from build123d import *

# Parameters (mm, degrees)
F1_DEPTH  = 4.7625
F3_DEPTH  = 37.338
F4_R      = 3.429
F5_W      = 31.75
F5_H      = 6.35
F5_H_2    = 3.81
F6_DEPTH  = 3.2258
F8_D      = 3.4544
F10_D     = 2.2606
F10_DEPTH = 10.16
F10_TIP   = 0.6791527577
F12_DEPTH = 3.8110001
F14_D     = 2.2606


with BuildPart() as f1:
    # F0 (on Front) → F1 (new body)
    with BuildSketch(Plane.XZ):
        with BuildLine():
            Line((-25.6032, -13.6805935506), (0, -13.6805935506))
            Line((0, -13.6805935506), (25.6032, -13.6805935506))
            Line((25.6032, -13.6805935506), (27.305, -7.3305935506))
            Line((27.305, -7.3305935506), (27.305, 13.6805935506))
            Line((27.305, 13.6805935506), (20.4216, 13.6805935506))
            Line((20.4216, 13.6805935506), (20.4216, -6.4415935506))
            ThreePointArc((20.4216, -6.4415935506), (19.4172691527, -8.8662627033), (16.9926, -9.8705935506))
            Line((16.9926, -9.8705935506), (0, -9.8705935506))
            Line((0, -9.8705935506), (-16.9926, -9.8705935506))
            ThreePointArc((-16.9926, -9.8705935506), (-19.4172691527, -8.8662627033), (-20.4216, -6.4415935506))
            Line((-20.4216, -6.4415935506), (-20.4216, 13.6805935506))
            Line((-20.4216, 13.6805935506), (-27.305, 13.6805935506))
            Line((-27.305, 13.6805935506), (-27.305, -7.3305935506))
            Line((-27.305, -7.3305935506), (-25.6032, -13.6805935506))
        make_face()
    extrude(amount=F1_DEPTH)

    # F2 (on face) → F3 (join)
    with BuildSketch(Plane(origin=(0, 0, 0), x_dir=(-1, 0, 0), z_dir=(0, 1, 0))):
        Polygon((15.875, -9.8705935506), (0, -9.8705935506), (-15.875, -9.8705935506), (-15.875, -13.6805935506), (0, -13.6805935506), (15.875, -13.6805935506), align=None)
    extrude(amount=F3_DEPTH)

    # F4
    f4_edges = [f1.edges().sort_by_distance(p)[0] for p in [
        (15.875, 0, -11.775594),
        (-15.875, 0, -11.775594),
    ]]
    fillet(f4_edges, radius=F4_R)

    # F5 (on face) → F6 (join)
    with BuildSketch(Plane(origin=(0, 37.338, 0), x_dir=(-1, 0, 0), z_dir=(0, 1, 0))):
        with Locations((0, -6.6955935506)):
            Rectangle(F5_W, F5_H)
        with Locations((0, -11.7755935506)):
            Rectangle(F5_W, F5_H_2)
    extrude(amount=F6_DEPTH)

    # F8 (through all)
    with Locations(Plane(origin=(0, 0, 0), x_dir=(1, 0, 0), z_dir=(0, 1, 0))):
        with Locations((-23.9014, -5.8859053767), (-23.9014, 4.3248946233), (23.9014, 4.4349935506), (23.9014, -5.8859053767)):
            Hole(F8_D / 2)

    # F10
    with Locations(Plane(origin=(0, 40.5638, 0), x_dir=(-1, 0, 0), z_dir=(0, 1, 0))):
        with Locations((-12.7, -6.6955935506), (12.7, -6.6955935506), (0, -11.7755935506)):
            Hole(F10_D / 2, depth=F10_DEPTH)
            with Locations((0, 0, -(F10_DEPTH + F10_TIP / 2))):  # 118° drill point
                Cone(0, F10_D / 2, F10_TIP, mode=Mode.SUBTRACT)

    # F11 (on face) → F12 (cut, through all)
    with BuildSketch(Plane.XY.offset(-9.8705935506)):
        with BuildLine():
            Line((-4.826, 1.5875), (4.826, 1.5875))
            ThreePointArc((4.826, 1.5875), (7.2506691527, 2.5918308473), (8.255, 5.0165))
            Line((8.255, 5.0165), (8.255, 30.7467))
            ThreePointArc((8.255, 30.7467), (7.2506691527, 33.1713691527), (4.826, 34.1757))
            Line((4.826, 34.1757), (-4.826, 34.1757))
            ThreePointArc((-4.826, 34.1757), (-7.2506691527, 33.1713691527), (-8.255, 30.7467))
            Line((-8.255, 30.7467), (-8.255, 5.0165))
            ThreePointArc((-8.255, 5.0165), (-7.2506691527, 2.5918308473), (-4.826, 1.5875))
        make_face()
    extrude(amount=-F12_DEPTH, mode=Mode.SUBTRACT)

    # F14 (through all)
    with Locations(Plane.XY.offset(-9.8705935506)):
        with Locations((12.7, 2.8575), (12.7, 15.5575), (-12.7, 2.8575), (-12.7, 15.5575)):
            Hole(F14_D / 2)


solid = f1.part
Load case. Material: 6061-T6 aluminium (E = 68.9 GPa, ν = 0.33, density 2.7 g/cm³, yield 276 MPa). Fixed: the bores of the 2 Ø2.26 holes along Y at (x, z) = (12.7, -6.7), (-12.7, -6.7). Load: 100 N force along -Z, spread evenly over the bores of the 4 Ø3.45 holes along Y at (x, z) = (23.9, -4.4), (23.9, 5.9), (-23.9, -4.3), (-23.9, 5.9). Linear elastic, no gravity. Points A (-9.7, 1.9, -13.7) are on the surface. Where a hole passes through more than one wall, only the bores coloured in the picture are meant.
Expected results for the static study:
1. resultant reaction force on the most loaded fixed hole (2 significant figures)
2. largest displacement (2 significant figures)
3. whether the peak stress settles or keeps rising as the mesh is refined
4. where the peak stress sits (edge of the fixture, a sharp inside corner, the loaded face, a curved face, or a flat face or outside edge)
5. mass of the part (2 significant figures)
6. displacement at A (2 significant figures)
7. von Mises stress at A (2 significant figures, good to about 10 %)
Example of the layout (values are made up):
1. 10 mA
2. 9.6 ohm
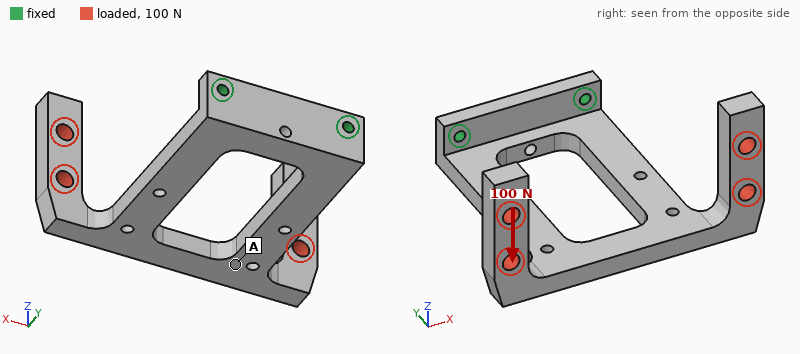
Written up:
1. 50 N
2. 0.91 mm
3. keeps rising
4. edge of the fixture
5. 16 g
6. 0.54 mm
7. 15 MPa
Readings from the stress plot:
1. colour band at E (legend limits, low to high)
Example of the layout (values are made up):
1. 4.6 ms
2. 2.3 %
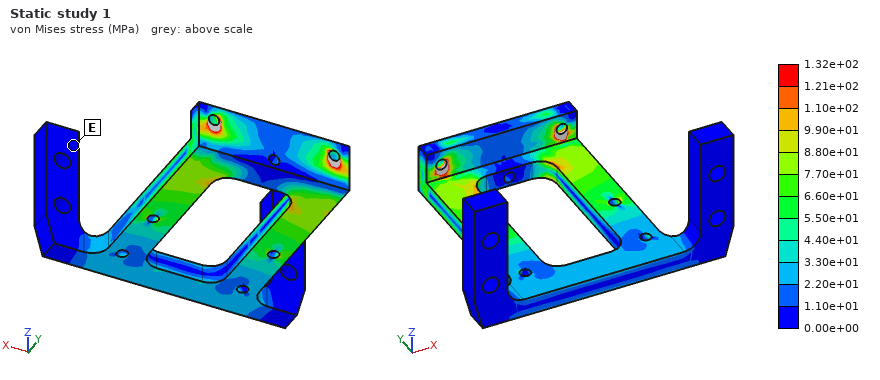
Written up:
1. 0.00e+00 to 1.10e+01 MPa
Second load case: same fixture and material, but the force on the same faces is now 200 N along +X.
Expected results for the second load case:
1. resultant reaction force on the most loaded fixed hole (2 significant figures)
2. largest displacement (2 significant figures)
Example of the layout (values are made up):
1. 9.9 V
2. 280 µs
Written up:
1. 320 N
2. 0.80 mm
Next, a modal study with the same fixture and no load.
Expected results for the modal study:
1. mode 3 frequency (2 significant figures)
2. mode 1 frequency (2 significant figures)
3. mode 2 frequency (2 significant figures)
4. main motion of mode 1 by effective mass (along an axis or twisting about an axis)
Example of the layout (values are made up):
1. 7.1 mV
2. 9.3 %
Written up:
1. 2100 Hz
2. 670 Hz
3. 1000 Hz
4. along Z
